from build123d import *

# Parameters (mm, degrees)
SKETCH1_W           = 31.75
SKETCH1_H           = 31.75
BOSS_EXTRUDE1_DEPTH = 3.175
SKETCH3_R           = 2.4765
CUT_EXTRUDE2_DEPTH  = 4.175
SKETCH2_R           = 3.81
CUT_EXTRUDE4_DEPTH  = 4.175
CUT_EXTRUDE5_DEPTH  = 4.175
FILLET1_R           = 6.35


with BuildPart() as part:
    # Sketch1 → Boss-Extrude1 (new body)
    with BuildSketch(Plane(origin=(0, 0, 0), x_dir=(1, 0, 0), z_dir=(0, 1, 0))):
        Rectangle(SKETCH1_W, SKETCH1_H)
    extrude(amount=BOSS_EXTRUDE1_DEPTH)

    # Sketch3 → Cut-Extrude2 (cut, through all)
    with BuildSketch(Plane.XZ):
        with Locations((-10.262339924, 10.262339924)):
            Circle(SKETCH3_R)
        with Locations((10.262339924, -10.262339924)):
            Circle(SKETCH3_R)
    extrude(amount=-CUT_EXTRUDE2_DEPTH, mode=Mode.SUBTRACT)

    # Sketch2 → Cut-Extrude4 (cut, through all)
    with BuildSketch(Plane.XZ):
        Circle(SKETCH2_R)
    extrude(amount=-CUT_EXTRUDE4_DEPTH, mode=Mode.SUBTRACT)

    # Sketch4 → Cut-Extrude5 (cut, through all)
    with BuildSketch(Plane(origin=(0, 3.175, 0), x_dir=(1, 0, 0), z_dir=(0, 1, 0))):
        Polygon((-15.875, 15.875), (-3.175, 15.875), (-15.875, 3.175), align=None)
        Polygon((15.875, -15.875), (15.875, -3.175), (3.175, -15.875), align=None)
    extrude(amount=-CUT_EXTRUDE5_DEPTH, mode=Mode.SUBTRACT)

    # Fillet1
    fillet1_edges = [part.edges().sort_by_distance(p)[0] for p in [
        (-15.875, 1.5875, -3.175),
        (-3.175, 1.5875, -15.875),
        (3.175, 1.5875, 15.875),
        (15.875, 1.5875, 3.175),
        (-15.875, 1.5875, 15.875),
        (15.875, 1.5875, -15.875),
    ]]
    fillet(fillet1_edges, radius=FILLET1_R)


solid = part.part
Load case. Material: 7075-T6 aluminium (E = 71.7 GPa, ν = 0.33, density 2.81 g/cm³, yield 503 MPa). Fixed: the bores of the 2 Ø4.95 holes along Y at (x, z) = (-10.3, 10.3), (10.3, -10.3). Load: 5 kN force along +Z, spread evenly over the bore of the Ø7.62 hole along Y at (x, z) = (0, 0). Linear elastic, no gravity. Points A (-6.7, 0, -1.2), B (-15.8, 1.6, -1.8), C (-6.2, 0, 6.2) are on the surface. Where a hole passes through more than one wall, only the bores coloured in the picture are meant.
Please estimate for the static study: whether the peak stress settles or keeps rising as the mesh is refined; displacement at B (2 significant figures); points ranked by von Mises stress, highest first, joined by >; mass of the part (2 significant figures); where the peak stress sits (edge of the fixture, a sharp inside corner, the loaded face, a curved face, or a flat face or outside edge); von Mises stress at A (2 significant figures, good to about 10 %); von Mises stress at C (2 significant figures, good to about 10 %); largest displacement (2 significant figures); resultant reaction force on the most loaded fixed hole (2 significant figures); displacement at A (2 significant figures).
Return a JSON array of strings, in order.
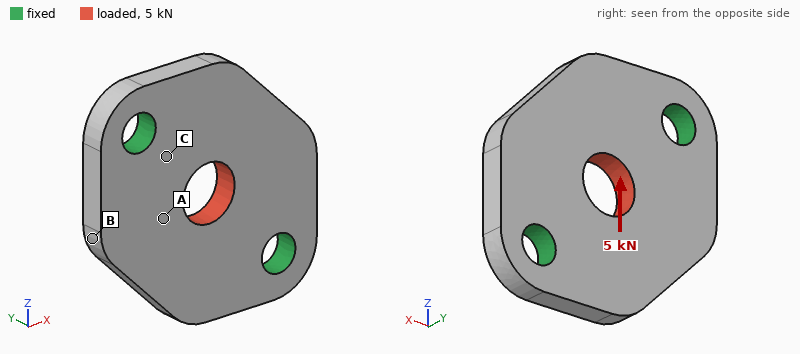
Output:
["keeps rising", "4.4 µm", "C > A > B", "6.6 g", "edge of the fixture", "49 MPa", "81 MPa", "18 µm", "2.5 kN", "12 µm"]
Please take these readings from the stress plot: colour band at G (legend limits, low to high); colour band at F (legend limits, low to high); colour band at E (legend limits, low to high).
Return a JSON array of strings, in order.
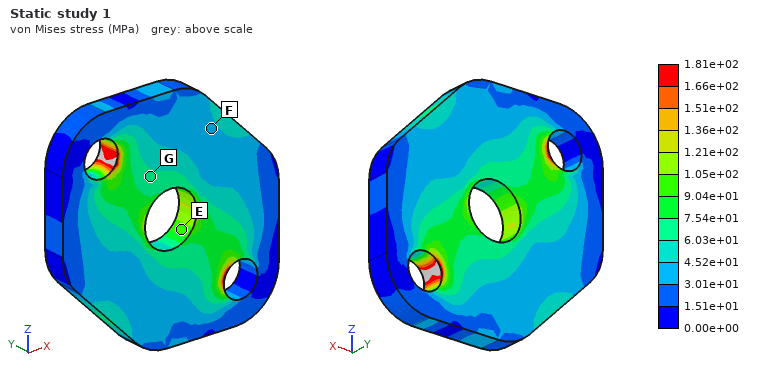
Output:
["6.03e+01 to 7.54e+01 MPa", "3.01e+01 to 4.52e+01 MPa", "9.04e+01 to 1.05e+02 MPa"]
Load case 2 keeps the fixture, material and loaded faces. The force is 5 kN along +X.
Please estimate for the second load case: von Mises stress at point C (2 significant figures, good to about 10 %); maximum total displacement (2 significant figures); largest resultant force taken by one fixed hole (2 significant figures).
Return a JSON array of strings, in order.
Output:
["81 MPa", "18 µm", "2.5 kN"]
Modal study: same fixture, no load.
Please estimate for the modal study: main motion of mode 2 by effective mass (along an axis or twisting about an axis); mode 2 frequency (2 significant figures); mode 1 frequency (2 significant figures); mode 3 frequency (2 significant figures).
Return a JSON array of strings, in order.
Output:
["along Y", "14 kHz", "12 kHz", "29 kHz"]
